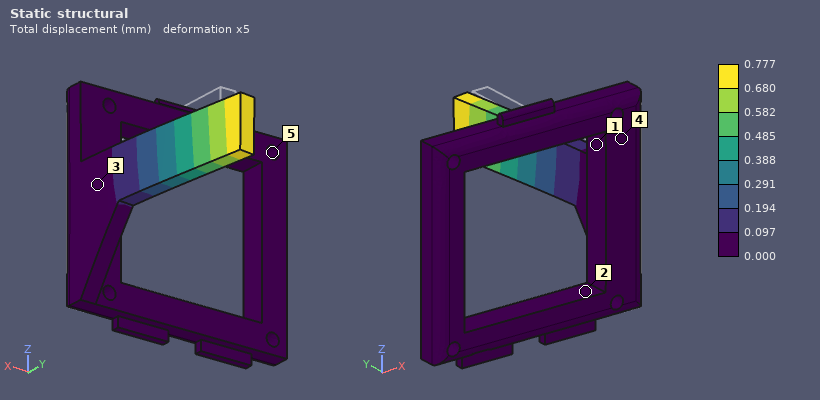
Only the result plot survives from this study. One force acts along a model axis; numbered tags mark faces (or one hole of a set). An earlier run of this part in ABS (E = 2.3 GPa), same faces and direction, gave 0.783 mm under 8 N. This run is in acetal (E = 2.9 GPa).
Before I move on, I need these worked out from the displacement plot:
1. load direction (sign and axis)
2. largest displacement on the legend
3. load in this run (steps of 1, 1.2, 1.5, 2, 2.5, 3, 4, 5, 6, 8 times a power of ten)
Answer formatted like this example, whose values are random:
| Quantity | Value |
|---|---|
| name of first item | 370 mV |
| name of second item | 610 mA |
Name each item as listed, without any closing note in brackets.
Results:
| Quantity | Value |
|---|---|
| load direction | -X |
| largest displacement on the legend | 0.777 mm |
| load in this run | 10 N |
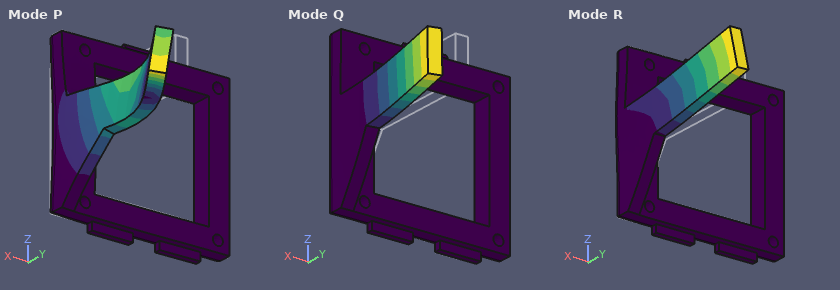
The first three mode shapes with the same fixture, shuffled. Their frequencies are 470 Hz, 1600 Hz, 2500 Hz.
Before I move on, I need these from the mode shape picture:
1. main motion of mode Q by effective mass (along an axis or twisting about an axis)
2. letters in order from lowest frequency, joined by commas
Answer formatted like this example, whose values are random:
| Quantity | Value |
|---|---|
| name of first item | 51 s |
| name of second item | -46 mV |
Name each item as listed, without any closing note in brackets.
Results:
| Quantity | Value |
|---|---|
| main motion of mode Q by effective mass | along X |
| letters in order from lowest frequency, joined by commas | Q, R, P |
